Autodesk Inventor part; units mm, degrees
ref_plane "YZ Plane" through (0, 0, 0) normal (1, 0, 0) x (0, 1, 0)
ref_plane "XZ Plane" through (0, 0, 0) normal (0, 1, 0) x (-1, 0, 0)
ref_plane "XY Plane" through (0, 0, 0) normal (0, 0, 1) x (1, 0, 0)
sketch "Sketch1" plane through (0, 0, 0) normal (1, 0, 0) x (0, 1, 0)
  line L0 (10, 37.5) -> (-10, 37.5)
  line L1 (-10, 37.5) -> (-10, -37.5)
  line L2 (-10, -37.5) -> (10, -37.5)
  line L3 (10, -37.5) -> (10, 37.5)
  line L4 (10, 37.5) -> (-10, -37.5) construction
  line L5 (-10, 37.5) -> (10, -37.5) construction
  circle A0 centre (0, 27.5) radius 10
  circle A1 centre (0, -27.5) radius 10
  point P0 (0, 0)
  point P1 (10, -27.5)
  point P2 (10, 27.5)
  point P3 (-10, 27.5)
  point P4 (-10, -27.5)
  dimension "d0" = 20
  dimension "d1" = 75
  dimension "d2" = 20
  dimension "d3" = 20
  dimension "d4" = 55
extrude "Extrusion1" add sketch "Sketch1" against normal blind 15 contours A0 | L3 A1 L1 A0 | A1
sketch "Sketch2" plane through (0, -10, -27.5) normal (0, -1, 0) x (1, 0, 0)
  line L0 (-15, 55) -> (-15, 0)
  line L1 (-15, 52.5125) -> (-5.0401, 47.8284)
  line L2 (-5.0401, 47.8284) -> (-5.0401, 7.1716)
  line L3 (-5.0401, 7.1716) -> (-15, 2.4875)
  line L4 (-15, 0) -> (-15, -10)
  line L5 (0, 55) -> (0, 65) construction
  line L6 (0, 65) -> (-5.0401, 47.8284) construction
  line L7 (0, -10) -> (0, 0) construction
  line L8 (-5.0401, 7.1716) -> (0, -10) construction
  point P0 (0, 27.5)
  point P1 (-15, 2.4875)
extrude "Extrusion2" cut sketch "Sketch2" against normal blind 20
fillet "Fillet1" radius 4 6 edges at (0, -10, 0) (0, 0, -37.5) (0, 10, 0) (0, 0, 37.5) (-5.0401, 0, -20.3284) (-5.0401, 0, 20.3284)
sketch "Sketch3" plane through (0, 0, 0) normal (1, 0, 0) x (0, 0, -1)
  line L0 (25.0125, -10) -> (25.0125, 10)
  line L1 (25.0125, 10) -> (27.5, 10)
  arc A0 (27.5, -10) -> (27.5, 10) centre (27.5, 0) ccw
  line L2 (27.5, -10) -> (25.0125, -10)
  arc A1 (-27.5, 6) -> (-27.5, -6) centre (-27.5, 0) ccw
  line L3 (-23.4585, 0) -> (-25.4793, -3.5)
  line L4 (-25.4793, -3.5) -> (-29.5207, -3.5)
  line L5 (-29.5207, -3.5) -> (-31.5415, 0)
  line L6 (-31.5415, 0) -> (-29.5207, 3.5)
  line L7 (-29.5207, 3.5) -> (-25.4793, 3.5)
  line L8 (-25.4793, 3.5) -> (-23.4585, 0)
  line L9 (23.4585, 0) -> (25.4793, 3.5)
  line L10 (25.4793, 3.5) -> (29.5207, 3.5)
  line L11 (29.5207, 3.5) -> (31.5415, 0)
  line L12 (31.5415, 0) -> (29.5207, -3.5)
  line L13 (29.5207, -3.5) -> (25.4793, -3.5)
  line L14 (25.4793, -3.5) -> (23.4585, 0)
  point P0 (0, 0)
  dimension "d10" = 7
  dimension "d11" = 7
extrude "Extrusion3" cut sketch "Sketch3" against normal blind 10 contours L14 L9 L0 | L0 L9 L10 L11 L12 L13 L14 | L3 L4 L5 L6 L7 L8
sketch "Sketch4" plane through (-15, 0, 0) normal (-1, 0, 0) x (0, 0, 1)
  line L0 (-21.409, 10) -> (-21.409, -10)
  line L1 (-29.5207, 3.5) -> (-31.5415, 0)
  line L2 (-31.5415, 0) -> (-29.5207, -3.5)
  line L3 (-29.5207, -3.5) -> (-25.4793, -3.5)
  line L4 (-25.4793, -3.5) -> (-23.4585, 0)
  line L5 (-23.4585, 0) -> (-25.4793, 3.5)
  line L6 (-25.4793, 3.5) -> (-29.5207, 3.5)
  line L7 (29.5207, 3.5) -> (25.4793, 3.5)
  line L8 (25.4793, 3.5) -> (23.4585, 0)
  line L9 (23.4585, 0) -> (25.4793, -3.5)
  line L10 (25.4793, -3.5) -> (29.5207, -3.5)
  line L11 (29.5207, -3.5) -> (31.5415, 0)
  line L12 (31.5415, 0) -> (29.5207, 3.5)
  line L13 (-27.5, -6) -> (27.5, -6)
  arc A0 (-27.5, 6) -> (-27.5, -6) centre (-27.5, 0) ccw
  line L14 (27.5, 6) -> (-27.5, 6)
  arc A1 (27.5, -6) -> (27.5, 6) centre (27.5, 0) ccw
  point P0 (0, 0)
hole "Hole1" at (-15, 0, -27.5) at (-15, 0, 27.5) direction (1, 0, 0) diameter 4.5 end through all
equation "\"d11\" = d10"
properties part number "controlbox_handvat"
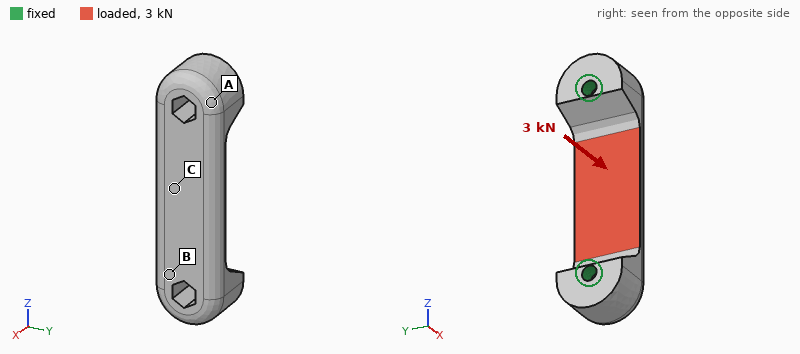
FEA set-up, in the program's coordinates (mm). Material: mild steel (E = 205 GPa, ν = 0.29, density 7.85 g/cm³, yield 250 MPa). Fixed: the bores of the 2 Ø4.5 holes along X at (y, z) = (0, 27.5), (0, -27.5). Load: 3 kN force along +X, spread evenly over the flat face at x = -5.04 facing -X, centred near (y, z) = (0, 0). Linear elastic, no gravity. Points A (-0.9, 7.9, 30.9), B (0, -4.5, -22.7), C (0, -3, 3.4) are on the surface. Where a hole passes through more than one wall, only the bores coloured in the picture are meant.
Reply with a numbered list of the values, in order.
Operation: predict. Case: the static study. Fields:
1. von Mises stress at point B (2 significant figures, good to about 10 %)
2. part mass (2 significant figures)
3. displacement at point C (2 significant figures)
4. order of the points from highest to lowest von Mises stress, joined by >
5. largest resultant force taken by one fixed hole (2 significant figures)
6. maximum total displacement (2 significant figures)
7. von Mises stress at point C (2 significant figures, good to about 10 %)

1. 60 MPa
2. 84 g
3. 29 µm
4. C > B > A
5. 2.3 kN
6. 32 µm
7. 110 MPa
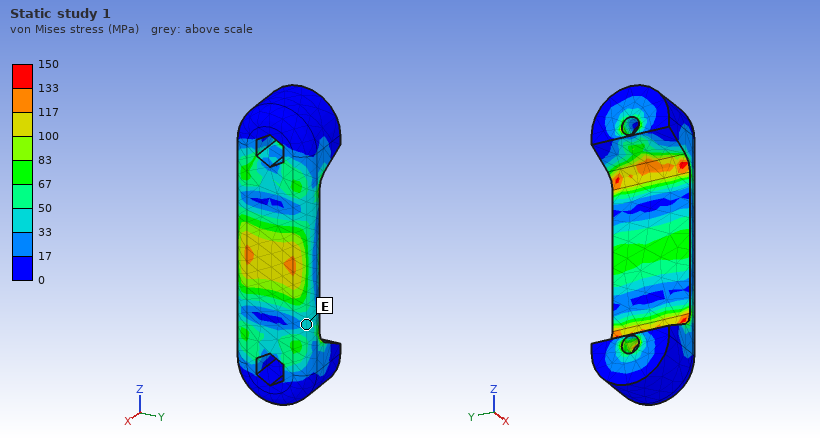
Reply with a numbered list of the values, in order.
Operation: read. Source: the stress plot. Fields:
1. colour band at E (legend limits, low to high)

1. 33 to 50 MPa
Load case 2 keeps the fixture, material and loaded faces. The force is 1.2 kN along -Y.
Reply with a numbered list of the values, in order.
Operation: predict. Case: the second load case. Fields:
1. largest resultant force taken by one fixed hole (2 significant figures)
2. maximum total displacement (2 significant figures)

1. 600 N
2. 7.8 µm
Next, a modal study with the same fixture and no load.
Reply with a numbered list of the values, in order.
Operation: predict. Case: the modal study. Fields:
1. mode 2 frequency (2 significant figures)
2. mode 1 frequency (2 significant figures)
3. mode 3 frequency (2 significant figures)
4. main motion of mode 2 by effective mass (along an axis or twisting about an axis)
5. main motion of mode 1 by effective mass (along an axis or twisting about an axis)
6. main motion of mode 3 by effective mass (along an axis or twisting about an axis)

1. 11 kHz
2. 10 kHz
3. 12 kHz
4. along X
5. along Y
6. along Z
